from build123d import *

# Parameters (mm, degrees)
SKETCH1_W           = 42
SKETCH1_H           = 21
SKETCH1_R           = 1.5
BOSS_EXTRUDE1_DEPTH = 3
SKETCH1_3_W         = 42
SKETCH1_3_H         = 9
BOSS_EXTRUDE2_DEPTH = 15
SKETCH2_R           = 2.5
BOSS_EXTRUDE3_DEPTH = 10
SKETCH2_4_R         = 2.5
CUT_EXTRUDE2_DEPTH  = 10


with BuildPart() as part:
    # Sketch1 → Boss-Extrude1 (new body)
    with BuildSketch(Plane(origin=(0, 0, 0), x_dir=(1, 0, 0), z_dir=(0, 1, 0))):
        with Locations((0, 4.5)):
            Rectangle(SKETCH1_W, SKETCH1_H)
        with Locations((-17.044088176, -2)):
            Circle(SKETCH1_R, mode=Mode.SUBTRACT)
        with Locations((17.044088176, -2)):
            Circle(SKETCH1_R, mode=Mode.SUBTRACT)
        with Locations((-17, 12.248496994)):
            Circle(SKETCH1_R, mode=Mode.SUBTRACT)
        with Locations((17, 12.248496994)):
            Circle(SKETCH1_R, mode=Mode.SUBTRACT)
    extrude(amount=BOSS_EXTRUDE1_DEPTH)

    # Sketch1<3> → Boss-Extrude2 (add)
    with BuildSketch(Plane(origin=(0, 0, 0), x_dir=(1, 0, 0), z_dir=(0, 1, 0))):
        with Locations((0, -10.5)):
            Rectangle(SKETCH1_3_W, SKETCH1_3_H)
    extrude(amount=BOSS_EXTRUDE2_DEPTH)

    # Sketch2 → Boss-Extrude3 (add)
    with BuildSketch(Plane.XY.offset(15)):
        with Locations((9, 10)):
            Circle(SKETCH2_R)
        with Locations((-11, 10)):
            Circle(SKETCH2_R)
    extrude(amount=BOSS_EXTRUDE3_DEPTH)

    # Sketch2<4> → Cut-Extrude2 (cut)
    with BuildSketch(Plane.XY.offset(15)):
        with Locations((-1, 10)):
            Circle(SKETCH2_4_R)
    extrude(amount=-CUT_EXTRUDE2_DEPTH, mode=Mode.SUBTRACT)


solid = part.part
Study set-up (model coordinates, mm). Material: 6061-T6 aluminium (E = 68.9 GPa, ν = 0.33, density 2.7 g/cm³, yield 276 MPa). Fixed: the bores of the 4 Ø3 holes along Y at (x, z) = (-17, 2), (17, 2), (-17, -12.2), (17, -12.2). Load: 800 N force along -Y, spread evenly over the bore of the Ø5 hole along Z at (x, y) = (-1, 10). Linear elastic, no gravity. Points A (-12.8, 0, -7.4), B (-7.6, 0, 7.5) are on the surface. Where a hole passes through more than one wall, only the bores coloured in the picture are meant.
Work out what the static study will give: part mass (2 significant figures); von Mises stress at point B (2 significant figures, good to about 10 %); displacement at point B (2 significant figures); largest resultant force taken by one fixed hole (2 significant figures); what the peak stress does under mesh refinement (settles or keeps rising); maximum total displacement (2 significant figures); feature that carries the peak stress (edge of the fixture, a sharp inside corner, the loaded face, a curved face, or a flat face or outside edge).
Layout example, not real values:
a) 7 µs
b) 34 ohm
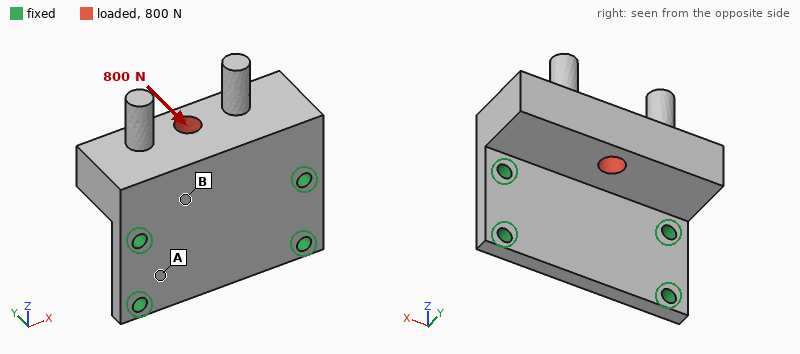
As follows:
a) 23 g
b) 27 MPa
c) 0.023 mm
d) 520 N
e) keeps rising
f) 0.11 mm
g) edge of the fixture
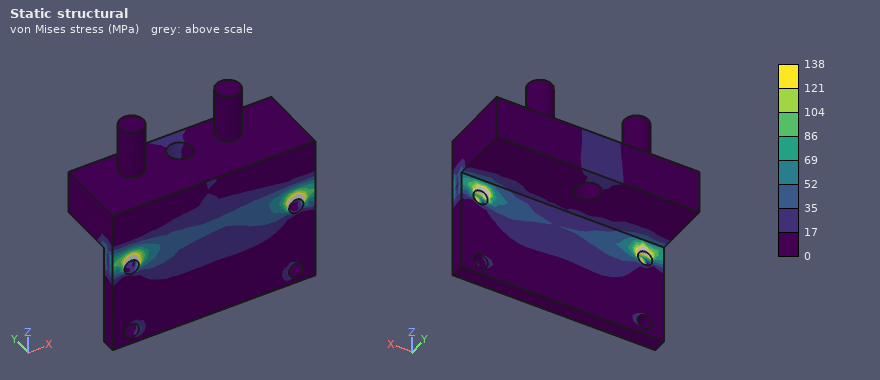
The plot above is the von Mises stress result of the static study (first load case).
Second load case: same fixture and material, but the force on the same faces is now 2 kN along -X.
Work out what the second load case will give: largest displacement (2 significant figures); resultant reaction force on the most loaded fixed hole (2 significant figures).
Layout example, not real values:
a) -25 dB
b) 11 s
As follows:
a) 21 µm
b) 1.1 kN
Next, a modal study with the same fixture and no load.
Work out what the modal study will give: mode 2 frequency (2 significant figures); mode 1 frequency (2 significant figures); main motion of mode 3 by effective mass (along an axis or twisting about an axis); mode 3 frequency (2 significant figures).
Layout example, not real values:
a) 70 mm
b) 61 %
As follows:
a) 12 kHz
b) 3800 Hz
c) along Y
d) 15 kHz
